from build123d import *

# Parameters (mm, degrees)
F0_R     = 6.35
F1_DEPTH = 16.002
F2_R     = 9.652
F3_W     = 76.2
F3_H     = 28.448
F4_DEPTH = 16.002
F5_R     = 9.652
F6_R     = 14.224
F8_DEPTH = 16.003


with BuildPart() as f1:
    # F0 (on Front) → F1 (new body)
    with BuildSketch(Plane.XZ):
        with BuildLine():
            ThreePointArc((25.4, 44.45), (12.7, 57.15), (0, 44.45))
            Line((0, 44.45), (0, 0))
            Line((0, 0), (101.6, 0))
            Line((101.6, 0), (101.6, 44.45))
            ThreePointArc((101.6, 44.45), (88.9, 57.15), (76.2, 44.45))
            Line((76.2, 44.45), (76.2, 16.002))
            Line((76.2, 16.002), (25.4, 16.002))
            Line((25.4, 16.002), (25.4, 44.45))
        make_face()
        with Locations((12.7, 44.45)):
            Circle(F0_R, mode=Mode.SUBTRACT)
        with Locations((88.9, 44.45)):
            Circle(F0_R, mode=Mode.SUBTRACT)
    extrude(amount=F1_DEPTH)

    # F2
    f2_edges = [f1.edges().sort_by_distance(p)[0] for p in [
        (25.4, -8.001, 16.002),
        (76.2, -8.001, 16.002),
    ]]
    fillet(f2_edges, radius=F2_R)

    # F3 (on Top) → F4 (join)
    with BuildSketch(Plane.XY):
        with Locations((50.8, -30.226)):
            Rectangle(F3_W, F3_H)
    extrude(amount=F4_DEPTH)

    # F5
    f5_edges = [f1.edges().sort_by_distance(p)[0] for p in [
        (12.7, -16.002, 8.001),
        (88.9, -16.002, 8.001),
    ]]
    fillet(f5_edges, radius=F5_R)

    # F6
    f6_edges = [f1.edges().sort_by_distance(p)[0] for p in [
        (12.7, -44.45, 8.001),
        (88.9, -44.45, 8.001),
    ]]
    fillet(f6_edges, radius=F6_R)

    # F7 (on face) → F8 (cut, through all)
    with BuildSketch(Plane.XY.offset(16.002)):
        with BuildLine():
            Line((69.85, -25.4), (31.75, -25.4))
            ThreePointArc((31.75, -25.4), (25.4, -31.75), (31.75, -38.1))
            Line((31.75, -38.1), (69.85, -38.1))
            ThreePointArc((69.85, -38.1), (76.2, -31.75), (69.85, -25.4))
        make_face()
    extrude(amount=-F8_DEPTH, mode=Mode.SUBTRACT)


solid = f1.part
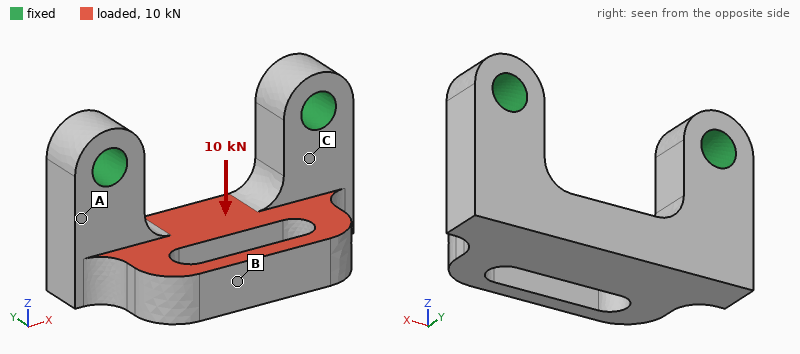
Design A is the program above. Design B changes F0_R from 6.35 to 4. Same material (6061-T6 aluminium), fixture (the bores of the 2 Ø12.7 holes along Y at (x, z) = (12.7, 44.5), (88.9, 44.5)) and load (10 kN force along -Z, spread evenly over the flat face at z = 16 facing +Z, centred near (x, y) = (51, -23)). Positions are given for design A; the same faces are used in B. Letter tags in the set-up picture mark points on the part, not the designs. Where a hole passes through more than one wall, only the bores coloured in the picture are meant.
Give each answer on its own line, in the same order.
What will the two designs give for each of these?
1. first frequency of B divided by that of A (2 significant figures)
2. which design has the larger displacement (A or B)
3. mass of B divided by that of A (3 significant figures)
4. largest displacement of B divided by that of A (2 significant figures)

0.90
B
1.03
1.1
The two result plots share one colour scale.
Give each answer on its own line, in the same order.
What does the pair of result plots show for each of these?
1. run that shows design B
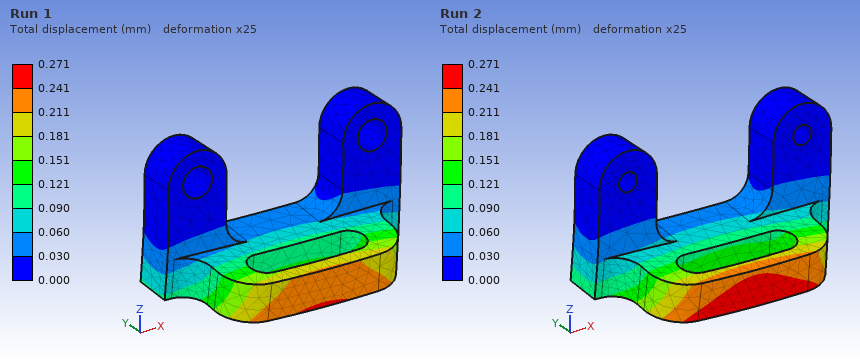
Run 2
